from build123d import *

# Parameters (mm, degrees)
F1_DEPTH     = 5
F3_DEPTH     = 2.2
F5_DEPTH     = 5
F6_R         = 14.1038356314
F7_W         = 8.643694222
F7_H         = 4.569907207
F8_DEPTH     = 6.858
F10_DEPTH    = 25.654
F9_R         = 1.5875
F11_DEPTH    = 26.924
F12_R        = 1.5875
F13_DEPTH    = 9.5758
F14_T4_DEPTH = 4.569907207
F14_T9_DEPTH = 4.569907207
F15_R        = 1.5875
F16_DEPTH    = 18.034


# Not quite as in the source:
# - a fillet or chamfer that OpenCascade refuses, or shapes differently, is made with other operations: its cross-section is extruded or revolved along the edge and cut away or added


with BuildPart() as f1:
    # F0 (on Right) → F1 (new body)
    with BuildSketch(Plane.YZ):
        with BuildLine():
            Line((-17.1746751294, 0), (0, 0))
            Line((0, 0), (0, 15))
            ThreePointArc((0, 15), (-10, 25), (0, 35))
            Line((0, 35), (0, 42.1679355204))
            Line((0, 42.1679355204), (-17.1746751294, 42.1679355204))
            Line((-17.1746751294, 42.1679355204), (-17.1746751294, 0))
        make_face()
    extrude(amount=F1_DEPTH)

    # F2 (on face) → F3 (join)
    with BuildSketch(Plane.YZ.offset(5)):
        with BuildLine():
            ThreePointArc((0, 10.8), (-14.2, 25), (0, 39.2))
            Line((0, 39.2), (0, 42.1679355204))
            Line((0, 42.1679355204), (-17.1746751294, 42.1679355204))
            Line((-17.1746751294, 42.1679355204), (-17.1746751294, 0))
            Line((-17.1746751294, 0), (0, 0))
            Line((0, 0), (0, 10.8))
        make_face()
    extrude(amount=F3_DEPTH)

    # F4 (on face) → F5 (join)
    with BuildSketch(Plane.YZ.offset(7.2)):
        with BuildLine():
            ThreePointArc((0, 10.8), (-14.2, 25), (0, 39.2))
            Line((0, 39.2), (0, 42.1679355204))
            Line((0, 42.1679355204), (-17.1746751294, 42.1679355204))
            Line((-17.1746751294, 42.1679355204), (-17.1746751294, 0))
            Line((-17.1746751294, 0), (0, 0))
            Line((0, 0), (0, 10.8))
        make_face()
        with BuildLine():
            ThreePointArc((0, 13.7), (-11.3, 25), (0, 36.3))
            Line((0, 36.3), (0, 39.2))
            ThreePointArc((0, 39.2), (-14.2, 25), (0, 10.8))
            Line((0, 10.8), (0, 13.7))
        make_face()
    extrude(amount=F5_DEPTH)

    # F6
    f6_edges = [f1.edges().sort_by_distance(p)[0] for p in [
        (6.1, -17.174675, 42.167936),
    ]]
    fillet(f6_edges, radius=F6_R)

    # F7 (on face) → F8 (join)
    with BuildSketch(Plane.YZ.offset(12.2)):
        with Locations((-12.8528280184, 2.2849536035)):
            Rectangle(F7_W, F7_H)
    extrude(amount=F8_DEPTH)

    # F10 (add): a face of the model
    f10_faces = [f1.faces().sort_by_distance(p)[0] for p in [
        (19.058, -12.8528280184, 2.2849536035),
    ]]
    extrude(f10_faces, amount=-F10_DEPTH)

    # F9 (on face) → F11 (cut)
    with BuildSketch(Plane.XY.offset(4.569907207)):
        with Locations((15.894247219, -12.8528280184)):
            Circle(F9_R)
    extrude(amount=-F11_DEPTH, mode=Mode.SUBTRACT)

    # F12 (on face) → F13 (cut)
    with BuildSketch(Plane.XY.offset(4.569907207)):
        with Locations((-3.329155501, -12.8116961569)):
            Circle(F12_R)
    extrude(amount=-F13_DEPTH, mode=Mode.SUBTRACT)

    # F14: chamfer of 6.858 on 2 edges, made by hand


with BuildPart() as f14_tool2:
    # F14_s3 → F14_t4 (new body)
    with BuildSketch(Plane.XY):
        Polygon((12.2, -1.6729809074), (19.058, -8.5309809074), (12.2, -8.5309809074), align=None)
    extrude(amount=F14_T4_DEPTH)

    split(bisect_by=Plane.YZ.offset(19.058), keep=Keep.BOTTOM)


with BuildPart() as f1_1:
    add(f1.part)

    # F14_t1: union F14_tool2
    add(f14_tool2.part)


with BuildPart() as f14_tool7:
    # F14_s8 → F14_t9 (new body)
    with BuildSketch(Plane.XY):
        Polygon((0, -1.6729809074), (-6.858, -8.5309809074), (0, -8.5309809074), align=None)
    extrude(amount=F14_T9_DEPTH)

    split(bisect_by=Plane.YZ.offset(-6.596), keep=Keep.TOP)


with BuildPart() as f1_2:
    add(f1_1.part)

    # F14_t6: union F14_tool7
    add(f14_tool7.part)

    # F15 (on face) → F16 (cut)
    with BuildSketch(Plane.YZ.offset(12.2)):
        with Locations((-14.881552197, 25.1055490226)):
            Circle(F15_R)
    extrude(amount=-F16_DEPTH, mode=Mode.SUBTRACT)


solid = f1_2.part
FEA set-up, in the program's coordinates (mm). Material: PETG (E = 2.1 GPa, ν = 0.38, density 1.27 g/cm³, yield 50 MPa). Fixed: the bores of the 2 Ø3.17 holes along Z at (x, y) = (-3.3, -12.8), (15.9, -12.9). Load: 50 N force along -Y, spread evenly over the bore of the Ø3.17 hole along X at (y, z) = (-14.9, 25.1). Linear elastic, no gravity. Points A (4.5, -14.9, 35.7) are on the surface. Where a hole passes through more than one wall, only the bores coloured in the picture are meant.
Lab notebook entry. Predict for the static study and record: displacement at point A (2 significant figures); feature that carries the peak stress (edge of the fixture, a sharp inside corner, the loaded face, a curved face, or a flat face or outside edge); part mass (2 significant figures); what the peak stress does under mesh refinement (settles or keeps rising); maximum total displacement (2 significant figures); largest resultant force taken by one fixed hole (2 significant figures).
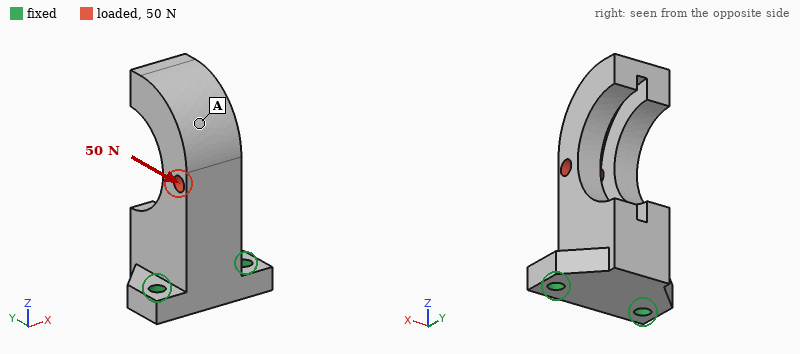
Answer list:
0.45 mm
edge of the fixture
8.1 g
keeps rising
0.58 mm
29 N
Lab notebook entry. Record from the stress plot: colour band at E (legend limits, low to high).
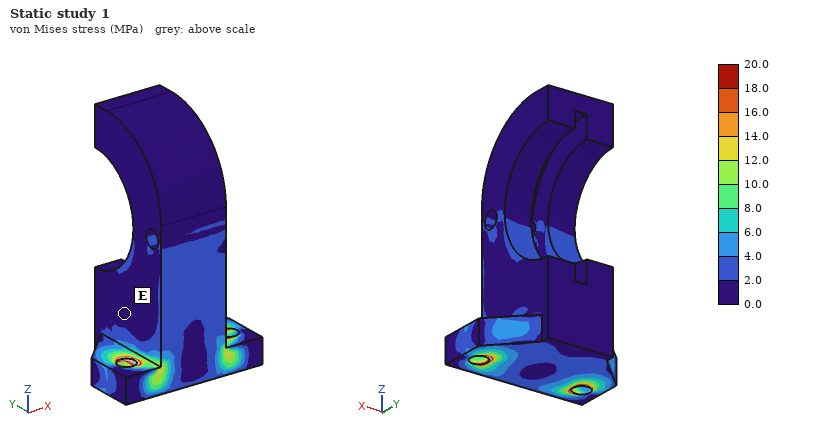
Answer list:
0.0 to 2.0 MPa
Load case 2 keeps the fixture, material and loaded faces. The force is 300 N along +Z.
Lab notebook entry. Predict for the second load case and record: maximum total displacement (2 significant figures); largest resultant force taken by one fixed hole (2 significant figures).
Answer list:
0.52 mm
160 N
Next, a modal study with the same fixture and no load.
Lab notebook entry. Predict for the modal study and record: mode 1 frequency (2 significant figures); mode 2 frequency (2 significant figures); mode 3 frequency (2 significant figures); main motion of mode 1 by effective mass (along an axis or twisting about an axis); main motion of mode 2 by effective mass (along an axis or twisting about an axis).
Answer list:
780 Hz
1200 Hz
2900 Hz
along Y
along X
